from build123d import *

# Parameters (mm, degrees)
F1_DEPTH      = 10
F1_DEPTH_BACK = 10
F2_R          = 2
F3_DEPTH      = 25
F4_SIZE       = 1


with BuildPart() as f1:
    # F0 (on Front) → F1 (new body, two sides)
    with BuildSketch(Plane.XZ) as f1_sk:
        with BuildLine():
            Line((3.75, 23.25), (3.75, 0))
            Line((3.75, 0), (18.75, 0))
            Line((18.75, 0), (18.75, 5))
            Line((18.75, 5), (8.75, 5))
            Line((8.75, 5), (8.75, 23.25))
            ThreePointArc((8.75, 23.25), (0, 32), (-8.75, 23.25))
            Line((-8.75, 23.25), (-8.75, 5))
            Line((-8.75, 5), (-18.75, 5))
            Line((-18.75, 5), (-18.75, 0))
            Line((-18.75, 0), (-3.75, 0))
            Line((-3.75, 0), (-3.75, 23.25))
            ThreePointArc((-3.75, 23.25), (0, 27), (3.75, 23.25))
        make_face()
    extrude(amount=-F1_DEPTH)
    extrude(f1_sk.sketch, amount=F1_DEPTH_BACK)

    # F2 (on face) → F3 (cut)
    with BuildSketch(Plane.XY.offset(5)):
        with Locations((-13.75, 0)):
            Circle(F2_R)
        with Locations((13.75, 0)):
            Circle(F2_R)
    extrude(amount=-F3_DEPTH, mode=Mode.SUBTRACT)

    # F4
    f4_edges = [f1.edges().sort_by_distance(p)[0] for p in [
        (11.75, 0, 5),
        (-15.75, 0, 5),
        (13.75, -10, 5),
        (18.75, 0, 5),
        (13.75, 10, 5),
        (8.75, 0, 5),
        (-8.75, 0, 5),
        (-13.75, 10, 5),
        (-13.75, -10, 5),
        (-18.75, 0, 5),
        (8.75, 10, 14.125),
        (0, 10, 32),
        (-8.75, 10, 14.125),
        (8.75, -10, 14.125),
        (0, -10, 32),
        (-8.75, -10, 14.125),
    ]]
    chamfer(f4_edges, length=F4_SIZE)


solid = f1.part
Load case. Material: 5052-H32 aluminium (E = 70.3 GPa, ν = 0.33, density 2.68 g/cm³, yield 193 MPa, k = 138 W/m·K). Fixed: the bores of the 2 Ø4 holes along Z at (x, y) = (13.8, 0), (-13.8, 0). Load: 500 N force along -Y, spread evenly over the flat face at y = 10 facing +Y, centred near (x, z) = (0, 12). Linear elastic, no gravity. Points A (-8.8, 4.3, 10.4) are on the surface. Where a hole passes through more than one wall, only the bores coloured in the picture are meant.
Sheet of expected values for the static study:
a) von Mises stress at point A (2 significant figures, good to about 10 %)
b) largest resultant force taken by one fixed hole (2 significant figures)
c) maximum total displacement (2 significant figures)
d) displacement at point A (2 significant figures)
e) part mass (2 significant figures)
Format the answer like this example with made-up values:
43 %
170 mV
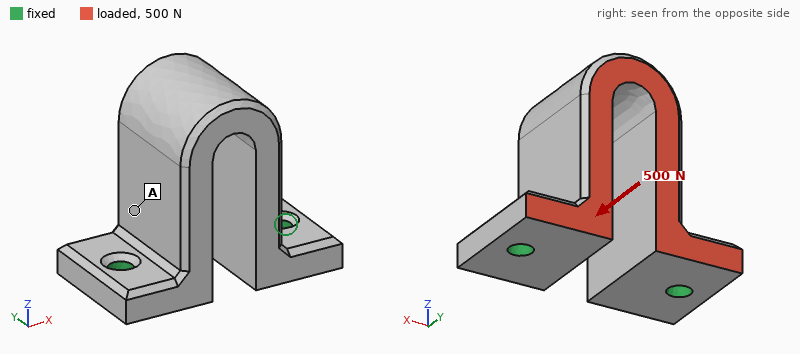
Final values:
6.5 MPa
250 N
34 µm
11 µm
22 g
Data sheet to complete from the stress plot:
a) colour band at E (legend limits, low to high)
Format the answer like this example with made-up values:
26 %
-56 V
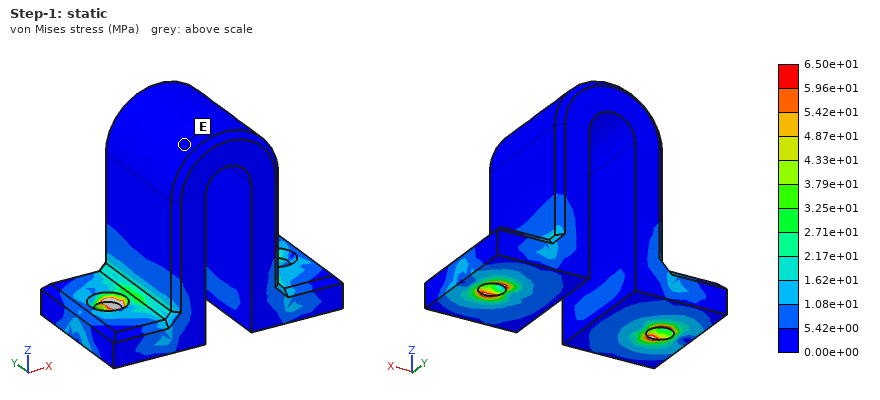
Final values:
0.00e+00 to 5.42e+00 MPa
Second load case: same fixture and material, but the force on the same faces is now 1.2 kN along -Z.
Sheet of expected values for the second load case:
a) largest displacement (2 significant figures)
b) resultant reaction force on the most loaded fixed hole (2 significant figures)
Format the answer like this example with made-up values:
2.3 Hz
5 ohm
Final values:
69 µm
610 N
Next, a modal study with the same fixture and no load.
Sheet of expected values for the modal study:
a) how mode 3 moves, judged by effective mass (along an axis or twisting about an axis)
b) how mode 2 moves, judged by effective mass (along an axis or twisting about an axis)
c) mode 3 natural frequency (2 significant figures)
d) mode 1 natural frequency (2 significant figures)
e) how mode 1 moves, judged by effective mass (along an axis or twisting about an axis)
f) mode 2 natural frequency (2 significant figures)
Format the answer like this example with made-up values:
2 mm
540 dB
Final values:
twisting about Z
along X
12 kHz
4600 Hz
along Y
7300 Hz
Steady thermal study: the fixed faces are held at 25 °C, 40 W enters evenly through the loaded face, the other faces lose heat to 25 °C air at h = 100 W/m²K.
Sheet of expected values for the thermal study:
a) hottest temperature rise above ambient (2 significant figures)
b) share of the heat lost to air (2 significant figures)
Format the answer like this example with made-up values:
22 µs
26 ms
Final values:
24 K
12 %
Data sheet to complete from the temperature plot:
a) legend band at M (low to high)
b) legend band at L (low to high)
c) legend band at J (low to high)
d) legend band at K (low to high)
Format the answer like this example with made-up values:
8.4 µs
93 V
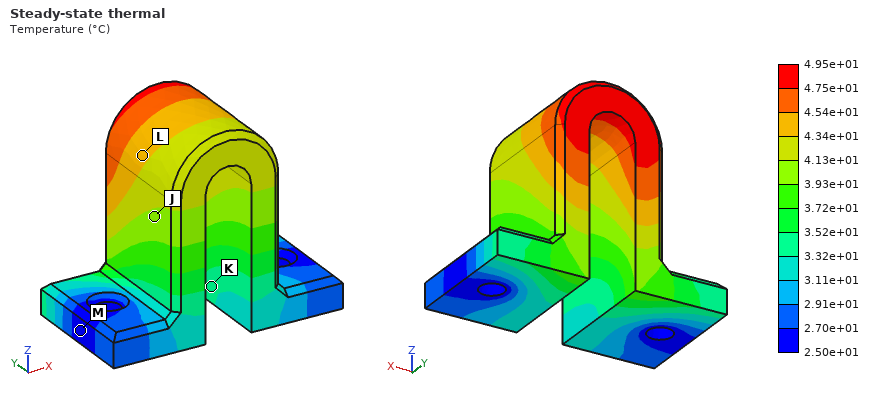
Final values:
2.50e+01 to 2.70e+01 °C
4.34e+01 to 4.54e+01 °C
3.93e+01 to 4.13e+01 °C
3.32e+01 to 3.52e+01 °C
